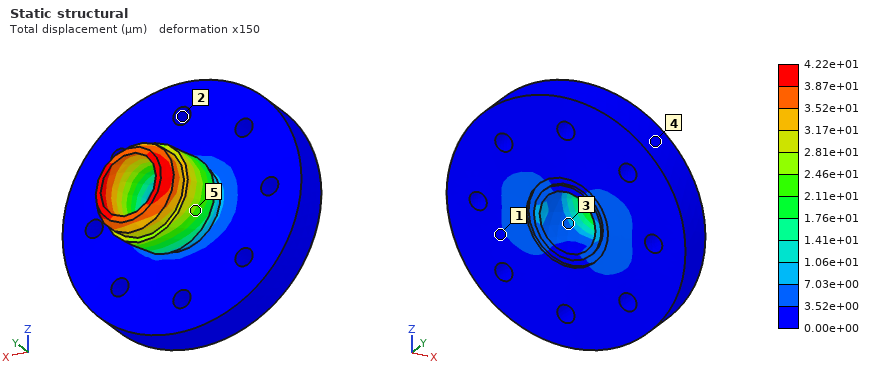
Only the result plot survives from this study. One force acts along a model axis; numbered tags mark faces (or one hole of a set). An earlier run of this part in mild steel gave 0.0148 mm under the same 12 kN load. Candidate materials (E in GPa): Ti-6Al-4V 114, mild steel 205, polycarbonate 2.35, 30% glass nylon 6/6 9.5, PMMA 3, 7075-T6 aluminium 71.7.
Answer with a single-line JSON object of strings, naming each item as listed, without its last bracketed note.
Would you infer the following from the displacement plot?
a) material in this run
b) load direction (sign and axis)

{"material in this run": "7075-T6 aluminium", "load direction": "+X"}
